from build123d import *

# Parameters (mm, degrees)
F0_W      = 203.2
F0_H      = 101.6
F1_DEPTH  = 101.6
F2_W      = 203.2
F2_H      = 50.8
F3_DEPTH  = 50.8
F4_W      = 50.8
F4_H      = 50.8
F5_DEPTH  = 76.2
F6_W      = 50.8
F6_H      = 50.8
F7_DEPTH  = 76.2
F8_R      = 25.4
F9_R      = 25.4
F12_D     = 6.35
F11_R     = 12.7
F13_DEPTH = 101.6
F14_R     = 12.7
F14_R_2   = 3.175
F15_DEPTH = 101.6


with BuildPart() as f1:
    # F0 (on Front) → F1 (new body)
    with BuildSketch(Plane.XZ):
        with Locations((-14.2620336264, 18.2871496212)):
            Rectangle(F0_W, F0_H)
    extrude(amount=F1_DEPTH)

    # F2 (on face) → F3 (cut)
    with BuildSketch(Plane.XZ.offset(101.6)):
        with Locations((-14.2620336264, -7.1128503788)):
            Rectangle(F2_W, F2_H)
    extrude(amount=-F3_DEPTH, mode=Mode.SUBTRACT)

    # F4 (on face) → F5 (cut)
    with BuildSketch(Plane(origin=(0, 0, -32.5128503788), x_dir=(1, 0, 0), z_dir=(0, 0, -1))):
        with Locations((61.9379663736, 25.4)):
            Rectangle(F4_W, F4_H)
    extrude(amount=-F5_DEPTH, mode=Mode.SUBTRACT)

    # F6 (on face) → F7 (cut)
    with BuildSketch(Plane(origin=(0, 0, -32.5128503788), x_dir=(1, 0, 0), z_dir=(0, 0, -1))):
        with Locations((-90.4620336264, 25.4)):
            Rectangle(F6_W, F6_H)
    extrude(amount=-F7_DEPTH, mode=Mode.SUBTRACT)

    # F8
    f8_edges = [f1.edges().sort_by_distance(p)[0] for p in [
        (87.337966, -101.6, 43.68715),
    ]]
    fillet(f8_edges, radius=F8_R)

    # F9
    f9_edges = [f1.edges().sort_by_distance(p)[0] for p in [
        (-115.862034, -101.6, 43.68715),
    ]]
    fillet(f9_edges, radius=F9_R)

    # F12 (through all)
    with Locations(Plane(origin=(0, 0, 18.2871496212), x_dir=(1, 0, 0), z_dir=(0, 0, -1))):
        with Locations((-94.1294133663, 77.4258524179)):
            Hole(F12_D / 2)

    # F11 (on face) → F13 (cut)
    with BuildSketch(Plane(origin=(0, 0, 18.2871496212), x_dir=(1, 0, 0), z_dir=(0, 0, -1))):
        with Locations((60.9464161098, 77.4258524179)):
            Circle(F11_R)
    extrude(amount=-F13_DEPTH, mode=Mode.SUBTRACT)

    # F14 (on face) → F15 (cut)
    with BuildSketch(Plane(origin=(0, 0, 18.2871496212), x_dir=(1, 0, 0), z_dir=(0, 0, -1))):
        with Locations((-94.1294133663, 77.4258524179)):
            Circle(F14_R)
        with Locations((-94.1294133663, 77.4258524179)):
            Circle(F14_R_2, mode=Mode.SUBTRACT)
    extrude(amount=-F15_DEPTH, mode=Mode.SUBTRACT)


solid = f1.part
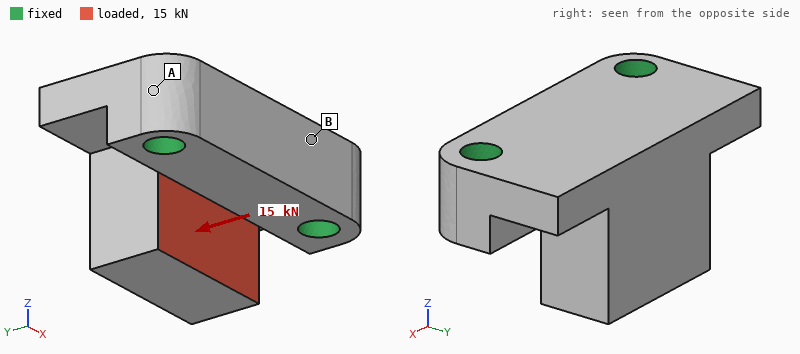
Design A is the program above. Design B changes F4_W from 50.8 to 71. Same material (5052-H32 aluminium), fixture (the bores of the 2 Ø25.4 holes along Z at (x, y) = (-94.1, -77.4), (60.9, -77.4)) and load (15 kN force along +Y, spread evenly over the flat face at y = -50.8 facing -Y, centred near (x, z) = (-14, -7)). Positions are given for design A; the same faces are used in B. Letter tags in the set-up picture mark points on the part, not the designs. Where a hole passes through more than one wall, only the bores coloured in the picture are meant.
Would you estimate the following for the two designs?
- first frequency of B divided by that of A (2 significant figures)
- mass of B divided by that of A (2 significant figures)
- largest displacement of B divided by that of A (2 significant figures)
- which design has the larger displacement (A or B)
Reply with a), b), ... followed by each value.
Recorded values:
a) 1.00
b) 0.96
c) 1.1
d) B
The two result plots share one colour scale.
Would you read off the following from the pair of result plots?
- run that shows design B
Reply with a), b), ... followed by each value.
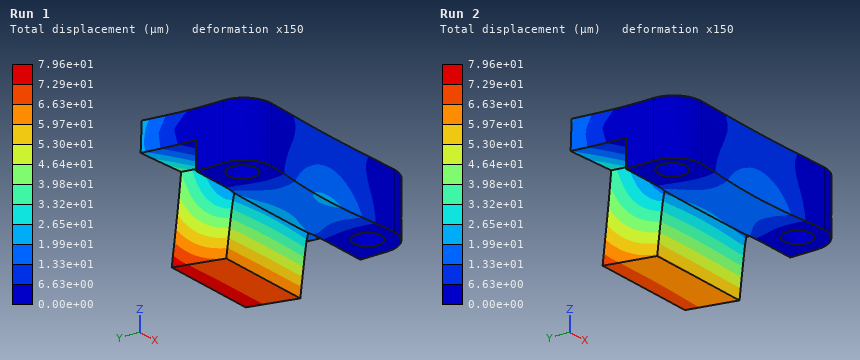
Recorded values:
a) Run 1
